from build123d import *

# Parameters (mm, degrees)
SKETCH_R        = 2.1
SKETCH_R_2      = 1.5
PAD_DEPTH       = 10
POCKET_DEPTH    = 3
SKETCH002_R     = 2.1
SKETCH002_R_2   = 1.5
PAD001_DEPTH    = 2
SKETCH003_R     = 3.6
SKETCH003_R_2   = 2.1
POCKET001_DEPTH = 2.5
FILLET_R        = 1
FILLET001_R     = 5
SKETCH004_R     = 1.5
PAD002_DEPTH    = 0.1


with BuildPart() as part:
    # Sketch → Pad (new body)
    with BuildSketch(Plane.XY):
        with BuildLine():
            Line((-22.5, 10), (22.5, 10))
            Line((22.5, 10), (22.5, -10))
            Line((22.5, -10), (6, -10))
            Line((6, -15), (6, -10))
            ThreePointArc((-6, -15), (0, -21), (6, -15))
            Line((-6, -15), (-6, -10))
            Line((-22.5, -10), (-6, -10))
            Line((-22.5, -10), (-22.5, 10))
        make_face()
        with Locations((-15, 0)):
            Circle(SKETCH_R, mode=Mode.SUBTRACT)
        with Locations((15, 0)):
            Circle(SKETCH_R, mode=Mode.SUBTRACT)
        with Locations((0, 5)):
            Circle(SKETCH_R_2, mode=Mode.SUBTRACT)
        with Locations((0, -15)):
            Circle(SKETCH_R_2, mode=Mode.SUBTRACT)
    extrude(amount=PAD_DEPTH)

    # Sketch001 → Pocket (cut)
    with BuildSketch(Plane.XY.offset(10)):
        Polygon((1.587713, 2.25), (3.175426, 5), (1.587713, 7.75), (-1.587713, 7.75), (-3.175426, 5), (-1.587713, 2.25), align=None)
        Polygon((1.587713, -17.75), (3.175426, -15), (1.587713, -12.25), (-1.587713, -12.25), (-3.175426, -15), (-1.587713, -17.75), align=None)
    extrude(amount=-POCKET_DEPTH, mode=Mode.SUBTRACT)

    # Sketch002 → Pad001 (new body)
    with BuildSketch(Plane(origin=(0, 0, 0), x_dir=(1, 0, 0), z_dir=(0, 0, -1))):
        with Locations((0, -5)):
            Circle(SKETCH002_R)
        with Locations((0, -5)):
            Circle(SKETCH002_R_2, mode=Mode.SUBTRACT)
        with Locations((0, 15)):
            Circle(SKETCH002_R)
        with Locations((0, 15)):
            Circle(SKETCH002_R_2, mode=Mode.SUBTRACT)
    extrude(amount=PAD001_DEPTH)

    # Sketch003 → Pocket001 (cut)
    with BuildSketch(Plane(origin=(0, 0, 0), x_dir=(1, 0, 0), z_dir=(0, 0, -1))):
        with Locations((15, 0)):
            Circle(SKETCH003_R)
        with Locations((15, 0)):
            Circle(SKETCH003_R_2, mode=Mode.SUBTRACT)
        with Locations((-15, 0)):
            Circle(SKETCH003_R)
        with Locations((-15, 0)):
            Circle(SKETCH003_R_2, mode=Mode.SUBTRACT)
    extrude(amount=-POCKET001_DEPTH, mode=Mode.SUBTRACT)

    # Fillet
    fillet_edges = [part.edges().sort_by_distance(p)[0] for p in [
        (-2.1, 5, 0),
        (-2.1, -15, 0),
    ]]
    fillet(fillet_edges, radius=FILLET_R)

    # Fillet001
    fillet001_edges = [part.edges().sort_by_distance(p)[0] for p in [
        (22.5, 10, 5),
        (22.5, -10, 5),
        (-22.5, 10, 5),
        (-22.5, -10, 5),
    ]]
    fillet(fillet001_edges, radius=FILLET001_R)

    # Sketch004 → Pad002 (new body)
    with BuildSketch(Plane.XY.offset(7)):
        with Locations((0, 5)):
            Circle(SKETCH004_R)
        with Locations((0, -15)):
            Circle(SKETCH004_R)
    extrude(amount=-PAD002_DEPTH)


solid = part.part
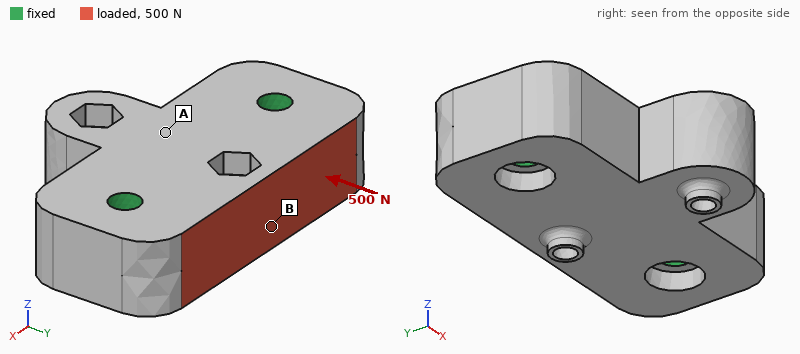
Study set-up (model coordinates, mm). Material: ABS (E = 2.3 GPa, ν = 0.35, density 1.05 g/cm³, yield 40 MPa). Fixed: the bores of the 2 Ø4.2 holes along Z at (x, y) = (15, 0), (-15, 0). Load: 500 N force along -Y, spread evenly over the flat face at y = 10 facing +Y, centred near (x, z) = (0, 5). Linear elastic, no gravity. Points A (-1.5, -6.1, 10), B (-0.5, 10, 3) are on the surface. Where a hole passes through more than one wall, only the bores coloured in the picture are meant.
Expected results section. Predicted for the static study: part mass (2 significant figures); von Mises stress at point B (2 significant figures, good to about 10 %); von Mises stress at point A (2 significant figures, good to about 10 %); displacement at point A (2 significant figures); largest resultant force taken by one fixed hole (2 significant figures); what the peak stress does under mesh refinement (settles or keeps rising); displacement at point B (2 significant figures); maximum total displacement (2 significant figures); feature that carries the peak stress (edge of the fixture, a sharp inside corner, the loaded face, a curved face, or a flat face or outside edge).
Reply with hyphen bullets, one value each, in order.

- 9.8 g
- 2.3 MPa
- 1.1 MPa
- 12 µm
- 250 N
- keeps rising
- 25 µm
- 28 µm
- edge of the fixture
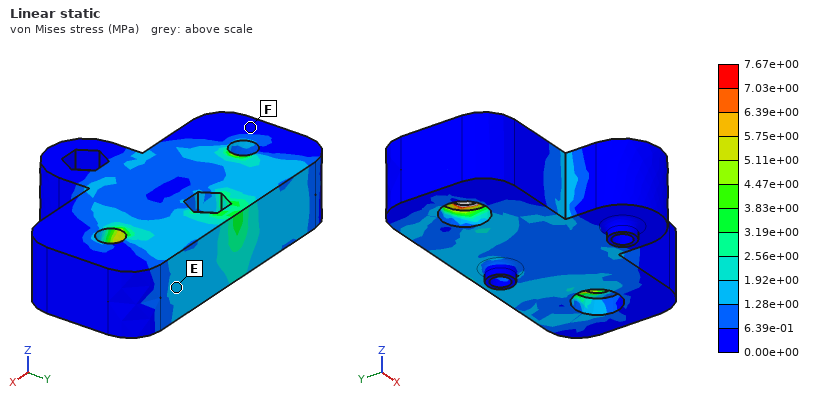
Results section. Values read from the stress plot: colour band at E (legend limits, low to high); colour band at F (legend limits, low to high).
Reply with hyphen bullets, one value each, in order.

- 1.28e+00 to 1.92e+00 MPa
- 0.00e+00 to 6.39e-01 MPa
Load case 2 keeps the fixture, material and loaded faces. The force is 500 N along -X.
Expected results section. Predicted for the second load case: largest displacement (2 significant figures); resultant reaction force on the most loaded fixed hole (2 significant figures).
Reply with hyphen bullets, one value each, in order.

- 24 µm
- 290 N
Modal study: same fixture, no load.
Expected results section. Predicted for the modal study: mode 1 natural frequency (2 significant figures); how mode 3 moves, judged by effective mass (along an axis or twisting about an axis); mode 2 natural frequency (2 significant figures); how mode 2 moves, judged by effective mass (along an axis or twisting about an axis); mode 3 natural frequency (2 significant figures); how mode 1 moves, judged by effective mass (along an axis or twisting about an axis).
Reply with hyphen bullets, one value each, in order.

- 4500 Hz
- along Y
- 8300 Hz
- along Z
- 9700 Hz
- along Z
